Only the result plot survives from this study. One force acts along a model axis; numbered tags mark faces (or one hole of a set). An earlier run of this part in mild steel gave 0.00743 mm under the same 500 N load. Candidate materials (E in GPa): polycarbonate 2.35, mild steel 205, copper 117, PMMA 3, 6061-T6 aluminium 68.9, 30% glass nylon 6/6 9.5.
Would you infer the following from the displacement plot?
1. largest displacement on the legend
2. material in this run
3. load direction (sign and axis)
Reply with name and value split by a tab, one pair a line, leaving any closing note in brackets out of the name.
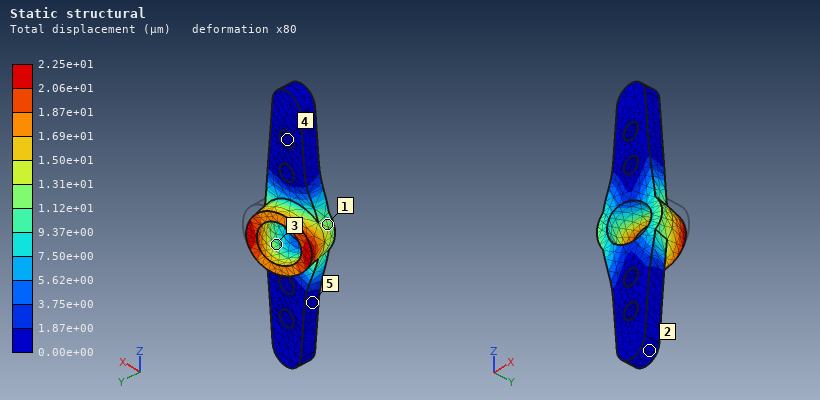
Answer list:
largest displacement on the legend	2.25e+01 µm
material in this run	6061-T6 aluminium
load direction	-X
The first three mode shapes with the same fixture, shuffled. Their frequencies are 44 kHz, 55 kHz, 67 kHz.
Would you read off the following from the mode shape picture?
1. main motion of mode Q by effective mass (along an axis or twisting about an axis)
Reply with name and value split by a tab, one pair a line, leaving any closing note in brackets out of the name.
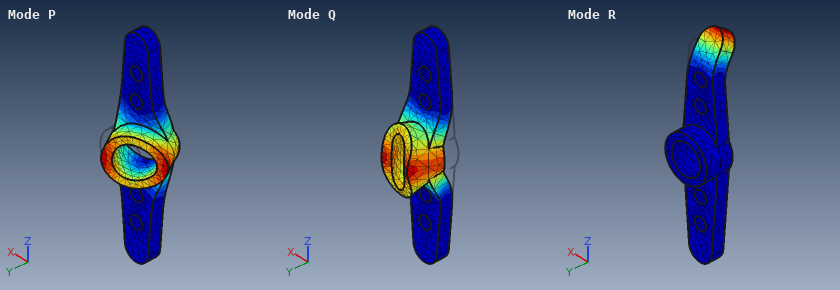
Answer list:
main motion of mode Q by effective mass	along Y
